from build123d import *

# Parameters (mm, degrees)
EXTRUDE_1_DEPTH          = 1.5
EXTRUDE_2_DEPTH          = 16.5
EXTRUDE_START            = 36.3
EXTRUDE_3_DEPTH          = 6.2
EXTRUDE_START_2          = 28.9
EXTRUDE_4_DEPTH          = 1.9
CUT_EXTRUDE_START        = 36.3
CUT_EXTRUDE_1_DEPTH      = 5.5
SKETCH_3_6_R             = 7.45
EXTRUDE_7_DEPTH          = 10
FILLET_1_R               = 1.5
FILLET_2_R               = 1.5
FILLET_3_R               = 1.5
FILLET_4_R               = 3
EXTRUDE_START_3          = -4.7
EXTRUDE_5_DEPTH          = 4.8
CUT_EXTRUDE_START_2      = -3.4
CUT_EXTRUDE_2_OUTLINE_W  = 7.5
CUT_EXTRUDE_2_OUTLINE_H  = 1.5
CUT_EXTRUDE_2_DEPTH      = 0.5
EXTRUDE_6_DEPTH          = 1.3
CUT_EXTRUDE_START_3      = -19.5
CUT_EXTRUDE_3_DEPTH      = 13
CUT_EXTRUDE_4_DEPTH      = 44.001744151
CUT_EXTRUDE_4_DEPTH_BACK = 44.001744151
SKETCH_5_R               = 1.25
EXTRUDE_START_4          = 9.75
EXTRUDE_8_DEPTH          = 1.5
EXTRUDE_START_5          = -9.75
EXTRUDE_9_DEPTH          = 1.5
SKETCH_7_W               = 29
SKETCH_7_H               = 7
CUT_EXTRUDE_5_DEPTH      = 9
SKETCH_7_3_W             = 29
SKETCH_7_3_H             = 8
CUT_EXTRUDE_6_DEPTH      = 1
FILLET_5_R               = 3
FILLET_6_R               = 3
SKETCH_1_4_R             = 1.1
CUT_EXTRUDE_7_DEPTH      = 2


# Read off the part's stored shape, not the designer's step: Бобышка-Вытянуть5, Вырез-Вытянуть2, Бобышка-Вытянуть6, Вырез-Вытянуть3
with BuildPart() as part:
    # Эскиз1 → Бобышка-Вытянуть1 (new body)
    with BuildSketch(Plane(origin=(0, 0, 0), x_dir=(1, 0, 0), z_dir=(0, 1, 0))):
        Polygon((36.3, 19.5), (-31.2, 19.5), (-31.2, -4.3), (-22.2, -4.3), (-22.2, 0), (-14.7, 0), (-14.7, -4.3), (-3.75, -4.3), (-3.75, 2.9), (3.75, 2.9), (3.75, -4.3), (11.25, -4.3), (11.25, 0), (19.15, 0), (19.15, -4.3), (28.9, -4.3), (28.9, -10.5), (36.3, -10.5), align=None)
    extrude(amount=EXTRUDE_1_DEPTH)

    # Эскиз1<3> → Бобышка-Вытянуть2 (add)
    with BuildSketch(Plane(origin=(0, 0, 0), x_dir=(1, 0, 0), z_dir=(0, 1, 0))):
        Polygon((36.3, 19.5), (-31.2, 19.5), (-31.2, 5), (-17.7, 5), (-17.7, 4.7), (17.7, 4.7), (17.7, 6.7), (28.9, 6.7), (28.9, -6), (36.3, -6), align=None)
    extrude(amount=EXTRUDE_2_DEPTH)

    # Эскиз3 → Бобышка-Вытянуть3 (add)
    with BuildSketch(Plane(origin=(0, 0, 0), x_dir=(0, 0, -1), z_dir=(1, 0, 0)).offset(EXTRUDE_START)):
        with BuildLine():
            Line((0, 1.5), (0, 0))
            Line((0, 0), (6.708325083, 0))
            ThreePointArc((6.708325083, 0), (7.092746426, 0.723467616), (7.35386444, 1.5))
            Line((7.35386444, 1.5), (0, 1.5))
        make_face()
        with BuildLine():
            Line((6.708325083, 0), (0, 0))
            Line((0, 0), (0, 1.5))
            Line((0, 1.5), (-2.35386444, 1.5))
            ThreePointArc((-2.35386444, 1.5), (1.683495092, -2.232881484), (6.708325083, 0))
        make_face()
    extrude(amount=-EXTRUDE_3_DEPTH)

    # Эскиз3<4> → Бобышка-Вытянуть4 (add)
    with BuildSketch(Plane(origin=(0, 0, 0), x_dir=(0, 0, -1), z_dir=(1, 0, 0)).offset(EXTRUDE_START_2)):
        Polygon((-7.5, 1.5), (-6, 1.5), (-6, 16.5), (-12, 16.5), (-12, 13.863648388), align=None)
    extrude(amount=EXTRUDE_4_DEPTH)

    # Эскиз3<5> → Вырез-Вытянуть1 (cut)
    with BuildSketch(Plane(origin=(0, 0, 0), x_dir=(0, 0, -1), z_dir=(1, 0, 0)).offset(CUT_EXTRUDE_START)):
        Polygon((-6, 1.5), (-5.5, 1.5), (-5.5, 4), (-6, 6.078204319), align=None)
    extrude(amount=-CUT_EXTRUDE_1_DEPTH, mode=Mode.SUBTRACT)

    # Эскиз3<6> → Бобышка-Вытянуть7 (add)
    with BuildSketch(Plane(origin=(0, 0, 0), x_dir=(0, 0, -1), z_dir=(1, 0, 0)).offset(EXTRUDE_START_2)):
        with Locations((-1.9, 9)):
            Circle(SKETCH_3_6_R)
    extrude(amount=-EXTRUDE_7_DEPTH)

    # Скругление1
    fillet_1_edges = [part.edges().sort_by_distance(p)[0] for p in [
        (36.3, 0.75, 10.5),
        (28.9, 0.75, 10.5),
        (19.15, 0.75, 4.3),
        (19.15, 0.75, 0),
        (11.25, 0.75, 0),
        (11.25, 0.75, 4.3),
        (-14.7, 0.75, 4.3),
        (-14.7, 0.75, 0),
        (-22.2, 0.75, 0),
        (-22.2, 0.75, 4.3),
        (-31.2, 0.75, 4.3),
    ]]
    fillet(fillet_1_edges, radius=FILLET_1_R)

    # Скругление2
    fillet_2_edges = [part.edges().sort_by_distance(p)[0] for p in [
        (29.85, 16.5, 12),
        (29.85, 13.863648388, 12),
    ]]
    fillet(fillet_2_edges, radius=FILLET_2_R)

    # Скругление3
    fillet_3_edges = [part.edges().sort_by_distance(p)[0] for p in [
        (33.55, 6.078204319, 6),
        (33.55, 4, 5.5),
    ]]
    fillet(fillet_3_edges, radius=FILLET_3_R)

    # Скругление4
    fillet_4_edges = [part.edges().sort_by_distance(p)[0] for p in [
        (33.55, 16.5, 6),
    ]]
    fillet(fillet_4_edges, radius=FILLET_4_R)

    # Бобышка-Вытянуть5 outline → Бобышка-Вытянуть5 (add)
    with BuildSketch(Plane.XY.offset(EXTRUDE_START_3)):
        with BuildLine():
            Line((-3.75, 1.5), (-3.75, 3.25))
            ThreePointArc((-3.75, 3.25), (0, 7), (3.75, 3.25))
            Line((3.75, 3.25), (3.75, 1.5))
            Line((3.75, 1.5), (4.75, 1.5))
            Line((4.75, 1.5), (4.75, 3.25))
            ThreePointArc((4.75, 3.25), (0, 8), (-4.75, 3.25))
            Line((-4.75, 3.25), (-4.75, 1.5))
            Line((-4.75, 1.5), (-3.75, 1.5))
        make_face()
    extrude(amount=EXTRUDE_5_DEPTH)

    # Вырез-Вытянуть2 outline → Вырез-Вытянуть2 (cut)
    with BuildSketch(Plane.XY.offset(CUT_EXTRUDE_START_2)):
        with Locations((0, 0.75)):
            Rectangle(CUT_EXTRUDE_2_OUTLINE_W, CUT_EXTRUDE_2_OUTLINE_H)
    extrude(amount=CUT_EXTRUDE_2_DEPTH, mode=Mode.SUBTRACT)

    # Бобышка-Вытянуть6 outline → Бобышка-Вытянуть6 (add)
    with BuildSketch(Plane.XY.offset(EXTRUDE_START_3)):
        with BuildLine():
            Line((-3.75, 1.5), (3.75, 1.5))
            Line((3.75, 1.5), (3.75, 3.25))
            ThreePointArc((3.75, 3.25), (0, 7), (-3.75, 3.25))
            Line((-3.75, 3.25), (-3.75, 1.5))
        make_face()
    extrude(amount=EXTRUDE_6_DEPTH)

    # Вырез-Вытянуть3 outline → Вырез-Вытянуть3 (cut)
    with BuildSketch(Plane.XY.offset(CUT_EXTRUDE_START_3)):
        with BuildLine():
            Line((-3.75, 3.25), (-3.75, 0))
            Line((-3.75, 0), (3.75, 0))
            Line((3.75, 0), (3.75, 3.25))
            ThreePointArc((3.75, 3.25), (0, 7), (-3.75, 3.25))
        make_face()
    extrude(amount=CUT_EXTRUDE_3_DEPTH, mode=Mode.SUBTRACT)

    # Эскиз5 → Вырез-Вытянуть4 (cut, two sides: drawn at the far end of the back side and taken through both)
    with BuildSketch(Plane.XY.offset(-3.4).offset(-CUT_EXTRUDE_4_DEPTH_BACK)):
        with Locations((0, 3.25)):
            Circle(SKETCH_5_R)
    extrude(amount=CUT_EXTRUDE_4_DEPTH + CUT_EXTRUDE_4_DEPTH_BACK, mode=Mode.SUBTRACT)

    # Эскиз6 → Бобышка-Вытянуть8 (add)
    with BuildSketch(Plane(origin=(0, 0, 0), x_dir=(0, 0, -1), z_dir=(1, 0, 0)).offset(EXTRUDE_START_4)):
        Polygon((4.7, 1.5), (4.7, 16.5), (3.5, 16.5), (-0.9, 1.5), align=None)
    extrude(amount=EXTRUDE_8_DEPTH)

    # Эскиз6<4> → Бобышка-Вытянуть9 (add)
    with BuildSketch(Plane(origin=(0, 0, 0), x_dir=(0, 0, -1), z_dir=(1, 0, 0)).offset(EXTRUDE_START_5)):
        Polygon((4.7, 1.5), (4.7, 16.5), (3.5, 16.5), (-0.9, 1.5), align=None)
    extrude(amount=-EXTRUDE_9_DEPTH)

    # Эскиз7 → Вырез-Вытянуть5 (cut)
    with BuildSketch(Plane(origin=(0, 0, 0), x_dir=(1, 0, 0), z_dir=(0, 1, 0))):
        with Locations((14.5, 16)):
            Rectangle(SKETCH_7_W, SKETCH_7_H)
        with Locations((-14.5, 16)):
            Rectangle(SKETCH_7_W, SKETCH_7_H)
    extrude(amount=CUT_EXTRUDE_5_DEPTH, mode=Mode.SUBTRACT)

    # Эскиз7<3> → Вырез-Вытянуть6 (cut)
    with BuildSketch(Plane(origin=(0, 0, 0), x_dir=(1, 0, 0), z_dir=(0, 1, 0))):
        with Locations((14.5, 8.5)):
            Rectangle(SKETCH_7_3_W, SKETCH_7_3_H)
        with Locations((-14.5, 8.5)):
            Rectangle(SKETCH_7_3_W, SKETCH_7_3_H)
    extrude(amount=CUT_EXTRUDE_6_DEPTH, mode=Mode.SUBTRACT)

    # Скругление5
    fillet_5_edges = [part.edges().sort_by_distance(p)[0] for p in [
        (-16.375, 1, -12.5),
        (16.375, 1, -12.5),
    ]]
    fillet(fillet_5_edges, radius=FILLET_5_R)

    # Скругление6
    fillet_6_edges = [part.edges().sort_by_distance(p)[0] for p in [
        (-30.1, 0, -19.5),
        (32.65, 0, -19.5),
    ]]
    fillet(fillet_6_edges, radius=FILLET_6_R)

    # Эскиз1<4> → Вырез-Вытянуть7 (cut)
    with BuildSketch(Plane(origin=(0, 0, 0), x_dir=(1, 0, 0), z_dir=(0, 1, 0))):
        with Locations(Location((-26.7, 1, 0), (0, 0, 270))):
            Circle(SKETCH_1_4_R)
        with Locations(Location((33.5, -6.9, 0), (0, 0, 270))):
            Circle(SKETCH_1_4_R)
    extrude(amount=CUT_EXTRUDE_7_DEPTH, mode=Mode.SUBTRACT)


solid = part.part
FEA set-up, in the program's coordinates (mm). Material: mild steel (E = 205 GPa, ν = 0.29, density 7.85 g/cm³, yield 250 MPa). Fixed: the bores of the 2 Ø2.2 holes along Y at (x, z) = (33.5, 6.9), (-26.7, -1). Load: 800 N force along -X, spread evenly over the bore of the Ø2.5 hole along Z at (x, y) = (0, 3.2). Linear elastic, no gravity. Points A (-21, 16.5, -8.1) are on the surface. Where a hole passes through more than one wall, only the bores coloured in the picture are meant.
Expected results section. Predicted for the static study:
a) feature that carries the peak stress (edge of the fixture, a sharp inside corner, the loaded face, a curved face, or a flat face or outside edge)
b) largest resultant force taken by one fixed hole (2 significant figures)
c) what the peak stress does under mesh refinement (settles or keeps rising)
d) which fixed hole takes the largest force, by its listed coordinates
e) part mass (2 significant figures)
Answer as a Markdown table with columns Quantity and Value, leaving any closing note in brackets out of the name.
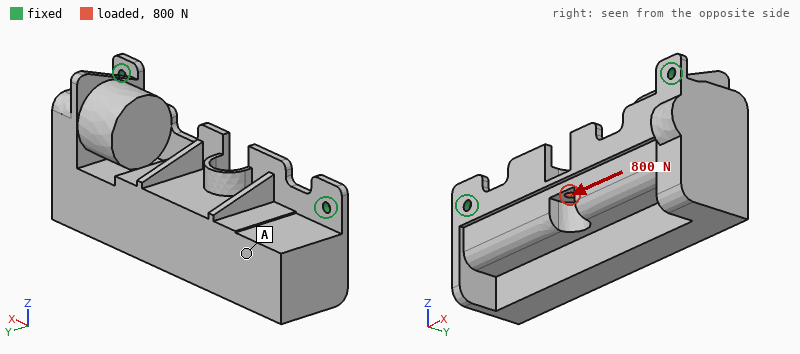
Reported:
| Quantity | Value |
|---|---|
| feature that carries the peak stress | edge of the fixture |
| largest resultant force taken by one fixed hole | 530 N |
| what the peak stress does under mesh refinement | keeps rising |
| which fixed hole takes the largest force, by its listed coordinates | (-26.7, -1) |
| part mass | 120 g |
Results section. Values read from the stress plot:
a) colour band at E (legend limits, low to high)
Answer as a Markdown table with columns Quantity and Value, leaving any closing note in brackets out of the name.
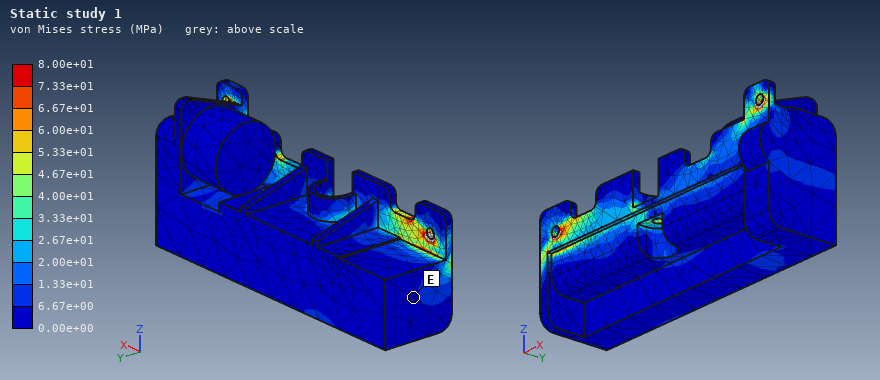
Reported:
| Quantity | Value |
|---|---|
| colour band at E | 0.00e+00 to 6.67e+00 MPa |
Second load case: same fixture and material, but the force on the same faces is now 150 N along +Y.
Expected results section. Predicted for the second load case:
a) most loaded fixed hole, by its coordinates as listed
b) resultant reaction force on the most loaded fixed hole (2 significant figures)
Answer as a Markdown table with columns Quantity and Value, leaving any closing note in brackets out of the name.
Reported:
| Quantity | Value |
|---|---|
| most loaded fixed hole, by its coordinates as listed | (-26.7, -1) |
| resultant reaction force on the most loaded fixed hole | 91 N |
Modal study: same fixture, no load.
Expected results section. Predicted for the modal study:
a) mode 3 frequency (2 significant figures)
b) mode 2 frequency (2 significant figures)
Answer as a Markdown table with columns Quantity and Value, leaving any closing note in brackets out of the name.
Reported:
| Quantity | Value |
|---|---|
| mode 3 frequency | 6100 Hz |
| mode 2 frequency | 4500 Hz |
